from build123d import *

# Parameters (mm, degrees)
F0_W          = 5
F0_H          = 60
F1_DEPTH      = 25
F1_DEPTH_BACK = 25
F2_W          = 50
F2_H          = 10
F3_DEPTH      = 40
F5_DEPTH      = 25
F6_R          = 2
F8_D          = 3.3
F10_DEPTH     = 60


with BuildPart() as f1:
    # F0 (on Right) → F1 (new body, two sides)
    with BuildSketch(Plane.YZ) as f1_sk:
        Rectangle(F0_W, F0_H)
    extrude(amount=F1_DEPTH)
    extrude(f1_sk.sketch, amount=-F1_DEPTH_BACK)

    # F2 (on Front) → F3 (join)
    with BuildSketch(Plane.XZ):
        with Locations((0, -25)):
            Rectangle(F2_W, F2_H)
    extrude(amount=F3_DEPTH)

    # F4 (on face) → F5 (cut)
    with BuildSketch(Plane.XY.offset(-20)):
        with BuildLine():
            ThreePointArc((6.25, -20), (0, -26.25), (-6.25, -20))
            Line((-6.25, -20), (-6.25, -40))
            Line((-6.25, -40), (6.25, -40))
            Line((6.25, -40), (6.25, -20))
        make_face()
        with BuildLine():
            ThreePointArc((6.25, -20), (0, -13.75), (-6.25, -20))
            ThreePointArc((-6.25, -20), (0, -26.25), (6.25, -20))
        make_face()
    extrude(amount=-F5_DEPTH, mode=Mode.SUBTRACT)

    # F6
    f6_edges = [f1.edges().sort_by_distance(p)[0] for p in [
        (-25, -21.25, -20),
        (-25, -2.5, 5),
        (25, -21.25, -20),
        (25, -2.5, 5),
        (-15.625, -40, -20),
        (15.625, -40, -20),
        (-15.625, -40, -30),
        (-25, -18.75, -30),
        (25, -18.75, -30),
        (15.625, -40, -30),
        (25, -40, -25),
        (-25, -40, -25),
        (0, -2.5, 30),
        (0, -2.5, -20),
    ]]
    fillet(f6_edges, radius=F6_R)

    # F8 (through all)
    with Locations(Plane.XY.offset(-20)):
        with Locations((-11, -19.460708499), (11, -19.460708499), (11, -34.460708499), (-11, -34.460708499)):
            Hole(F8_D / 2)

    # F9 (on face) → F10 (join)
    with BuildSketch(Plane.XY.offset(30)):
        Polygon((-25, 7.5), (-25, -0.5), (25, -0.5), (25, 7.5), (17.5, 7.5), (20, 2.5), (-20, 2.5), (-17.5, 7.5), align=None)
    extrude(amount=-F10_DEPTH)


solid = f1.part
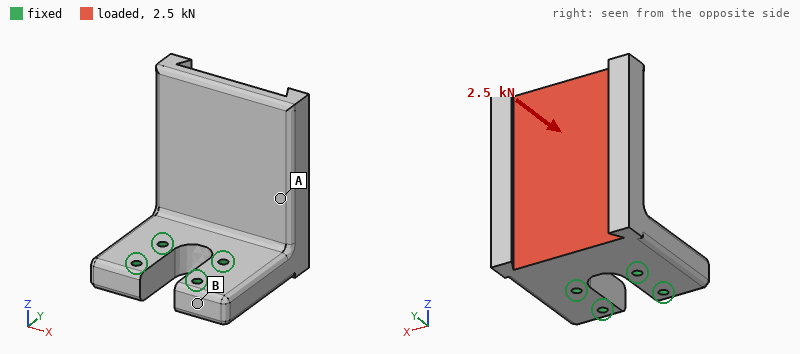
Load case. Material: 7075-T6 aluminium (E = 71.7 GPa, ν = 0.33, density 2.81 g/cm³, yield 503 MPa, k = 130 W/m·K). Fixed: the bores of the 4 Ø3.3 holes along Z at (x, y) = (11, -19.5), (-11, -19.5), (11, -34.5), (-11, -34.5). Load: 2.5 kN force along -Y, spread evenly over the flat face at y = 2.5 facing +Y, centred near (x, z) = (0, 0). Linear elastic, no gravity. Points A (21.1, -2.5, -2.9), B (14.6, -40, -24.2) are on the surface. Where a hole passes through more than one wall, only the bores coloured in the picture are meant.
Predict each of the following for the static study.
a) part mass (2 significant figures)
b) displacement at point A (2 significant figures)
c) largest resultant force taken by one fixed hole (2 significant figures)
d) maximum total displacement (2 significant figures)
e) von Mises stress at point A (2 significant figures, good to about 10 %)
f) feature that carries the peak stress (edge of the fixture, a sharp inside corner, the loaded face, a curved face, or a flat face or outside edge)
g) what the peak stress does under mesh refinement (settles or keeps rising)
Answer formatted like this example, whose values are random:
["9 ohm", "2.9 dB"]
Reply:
["95 g", "0.20 mm", "1.3 kN", "0.67 mm", "51 MPa", "edge of the fixture", "keeps rising"]
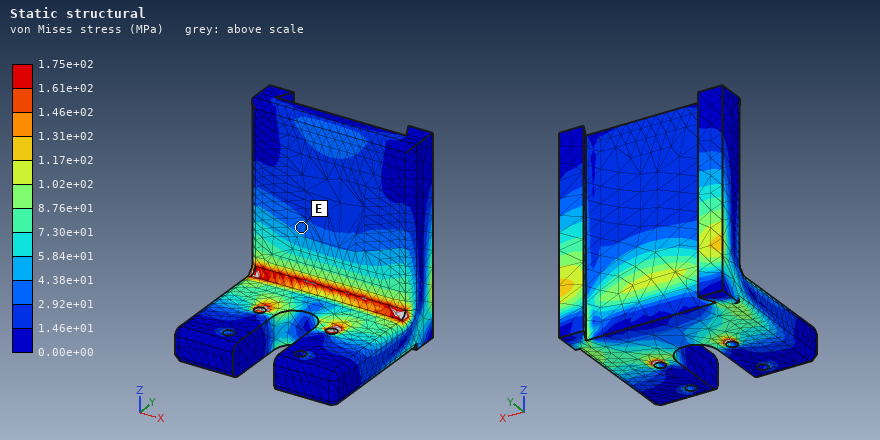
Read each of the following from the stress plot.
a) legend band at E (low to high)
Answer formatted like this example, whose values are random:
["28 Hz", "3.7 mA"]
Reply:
["2.92e+01 to 4.38e+01 MPa"]
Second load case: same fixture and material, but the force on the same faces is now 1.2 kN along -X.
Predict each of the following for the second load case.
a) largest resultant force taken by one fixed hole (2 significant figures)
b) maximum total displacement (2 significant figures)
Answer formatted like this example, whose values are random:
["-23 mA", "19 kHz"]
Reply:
["1.4 kN", "67 µm"]
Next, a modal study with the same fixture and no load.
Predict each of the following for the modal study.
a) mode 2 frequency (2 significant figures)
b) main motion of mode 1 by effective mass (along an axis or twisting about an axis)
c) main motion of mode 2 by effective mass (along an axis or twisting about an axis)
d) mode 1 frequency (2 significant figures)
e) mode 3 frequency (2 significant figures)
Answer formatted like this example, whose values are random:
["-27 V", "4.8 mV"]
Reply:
["3000 Hz", "along Y", "along X", "1700 Hz", "3800 Hz"]
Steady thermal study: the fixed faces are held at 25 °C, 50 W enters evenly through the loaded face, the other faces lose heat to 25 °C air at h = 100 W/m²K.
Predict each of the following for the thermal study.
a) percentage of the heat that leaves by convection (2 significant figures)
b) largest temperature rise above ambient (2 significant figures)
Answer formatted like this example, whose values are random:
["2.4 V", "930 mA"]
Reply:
["31 %", "33 K"]
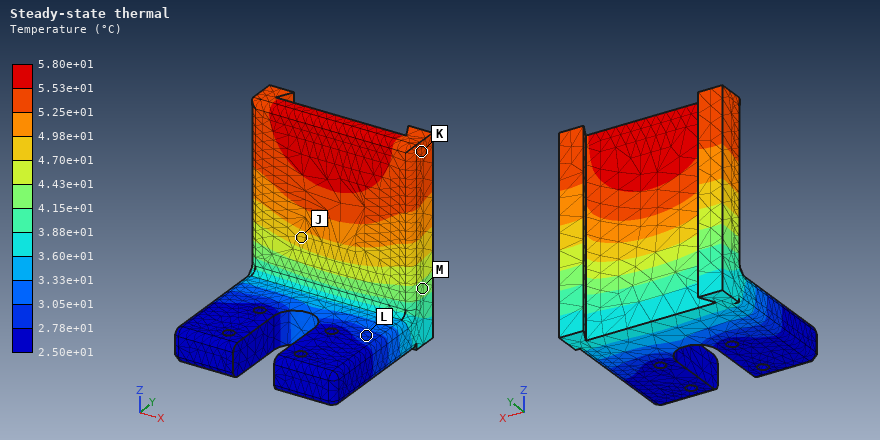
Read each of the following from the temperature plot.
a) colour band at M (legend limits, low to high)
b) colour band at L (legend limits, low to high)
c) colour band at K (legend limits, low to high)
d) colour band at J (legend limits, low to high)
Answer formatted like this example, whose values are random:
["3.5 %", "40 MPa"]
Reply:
["4.15e+01 to 4.43e+01 °C", "2.78e+01 to 3.05e+01 °C", "5.25e+01 to 5.53e+01 °C", "4.70e+01 to 4.98e+01 °C"]
